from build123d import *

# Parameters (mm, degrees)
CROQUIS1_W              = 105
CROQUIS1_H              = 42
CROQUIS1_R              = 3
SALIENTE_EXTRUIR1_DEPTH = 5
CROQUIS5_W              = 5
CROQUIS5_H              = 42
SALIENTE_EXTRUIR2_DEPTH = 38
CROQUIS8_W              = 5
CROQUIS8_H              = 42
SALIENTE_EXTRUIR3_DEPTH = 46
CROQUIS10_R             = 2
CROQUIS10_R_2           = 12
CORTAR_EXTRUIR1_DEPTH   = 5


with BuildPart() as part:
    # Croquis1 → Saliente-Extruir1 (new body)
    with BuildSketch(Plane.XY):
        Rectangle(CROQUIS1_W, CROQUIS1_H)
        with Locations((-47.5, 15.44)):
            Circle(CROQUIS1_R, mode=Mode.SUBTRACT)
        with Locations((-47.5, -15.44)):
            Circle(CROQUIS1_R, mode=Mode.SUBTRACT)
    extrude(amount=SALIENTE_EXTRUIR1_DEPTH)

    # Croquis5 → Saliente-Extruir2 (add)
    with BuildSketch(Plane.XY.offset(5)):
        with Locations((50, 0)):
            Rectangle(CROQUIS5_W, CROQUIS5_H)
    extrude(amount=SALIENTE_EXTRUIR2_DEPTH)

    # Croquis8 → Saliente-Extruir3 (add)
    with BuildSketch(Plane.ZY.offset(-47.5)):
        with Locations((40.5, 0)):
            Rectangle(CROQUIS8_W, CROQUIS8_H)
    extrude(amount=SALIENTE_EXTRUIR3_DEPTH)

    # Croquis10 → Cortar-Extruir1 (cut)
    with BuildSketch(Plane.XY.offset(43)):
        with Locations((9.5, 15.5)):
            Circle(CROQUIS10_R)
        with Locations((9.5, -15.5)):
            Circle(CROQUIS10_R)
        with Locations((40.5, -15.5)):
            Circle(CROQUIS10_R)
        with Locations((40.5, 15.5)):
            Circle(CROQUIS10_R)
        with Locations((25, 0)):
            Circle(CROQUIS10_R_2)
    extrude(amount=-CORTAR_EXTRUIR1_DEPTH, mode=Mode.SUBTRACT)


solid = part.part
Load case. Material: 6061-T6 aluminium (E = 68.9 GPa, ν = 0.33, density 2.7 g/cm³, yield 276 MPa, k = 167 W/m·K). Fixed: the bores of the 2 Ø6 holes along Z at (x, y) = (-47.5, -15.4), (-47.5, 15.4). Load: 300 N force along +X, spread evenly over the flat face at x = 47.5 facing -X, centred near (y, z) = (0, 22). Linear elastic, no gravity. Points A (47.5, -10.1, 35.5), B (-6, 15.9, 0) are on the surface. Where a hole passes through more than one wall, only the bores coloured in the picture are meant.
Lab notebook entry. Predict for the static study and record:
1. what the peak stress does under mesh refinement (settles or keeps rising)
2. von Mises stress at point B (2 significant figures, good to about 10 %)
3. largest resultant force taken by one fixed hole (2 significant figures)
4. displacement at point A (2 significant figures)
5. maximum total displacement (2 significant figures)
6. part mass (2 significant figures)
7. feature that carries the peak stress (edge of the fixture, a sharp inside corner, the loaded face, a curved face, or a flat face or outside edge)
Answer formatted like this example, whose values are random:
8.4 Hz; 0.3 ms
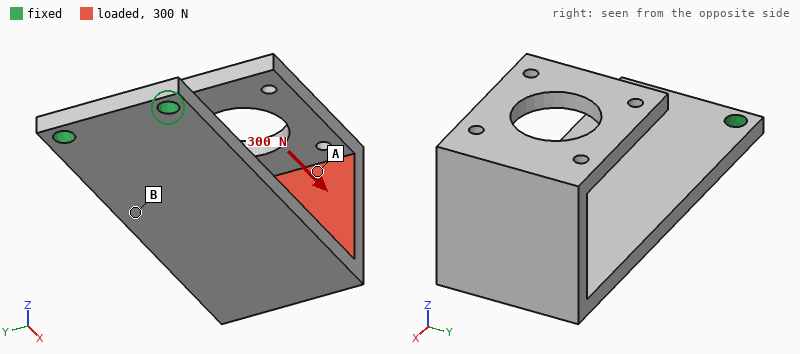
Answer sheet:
keeps rising; 31 MPa; 150 N; 1.1 mm; 1.2 mm; 100 g; edge of the fixture
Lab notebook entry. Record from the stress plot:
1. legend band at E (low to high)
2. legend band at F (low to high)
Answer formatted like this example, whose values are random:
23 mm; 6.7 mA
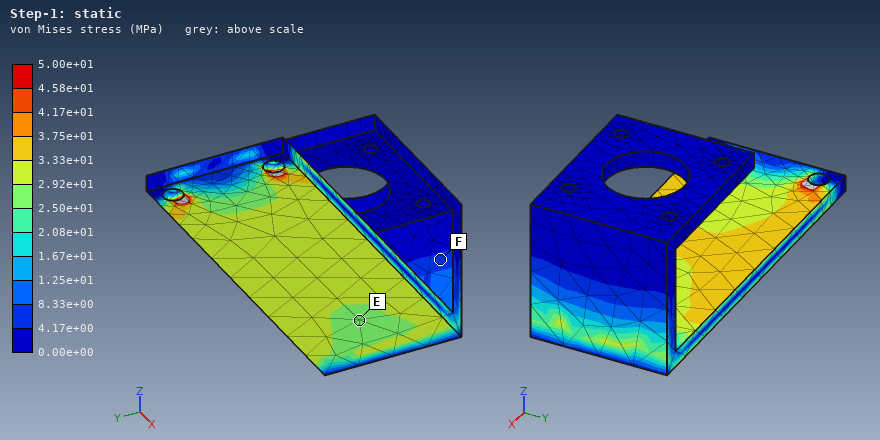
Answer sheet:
2.50e+01 to 2.92e+01 MPa; 4.17e+00 to 8.33e+00 MPa
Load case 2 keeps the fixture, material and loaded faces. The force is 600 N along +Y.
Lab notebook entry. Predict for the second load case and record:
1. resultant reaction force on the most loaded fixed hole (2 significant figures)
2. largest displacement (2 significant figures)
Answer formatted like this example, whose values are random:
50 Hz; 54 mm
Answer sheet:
1.8 kN; 1.1 mm
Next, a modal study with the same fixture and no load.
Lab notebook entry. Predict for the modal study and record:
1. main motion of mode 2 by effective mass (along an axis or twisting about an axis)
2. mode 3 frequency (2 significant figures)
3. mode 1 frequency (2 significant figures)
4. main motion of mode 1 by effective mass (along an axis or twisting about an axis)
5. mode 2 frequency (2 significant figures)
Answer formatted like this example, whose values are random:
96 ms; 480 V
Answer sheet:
along Y; 570 Hz; 220 Hz; along Z; 490 Hz
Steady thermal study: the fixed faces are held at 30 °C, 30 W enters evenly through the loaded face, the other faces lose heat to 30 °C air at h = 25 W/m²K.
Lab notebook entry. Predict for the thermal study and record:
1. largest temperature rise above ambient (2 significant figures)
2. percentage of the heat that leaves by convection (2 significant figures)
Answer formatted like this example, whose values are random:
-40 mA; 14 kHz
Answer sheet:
58 K; 47 %
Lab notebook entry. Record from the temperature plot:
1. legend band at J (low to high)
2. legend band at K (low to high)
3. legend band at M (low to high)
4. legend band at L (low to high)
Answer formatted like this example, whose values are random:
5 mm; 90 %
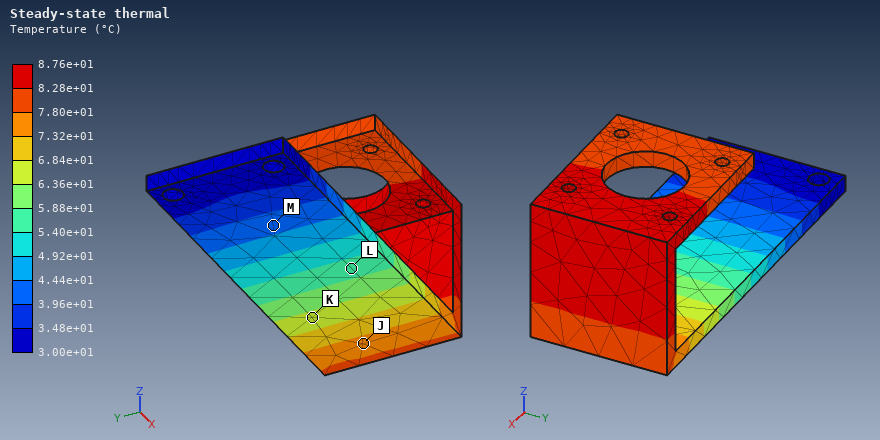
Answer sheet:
7.32e+01 to 7.80e+01 °C; 6.36e+01 to 6.84e+01 °C; 3.96e+01 to 4.44e+01 °C; 5.40e+01 to 5.88e+01 °C
